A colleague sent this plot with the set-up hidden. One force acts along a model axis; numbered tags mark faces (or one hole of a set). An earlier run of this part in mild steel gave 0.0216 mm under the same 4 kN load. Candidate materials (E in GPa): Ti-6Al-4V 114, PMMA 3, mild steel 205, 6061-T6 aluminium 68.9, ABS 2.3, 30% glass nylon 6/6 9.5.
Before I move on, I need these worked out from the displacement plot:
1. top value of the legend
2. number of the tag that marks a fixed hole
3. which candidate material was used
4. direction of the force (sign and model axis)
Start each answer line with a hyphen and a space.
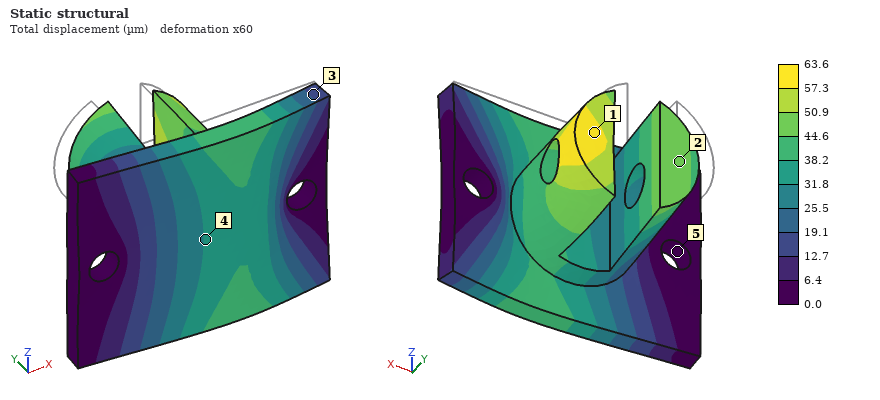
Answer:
- 63.6 µm
- 5
- 6061-T6 aluminium
- -Y
